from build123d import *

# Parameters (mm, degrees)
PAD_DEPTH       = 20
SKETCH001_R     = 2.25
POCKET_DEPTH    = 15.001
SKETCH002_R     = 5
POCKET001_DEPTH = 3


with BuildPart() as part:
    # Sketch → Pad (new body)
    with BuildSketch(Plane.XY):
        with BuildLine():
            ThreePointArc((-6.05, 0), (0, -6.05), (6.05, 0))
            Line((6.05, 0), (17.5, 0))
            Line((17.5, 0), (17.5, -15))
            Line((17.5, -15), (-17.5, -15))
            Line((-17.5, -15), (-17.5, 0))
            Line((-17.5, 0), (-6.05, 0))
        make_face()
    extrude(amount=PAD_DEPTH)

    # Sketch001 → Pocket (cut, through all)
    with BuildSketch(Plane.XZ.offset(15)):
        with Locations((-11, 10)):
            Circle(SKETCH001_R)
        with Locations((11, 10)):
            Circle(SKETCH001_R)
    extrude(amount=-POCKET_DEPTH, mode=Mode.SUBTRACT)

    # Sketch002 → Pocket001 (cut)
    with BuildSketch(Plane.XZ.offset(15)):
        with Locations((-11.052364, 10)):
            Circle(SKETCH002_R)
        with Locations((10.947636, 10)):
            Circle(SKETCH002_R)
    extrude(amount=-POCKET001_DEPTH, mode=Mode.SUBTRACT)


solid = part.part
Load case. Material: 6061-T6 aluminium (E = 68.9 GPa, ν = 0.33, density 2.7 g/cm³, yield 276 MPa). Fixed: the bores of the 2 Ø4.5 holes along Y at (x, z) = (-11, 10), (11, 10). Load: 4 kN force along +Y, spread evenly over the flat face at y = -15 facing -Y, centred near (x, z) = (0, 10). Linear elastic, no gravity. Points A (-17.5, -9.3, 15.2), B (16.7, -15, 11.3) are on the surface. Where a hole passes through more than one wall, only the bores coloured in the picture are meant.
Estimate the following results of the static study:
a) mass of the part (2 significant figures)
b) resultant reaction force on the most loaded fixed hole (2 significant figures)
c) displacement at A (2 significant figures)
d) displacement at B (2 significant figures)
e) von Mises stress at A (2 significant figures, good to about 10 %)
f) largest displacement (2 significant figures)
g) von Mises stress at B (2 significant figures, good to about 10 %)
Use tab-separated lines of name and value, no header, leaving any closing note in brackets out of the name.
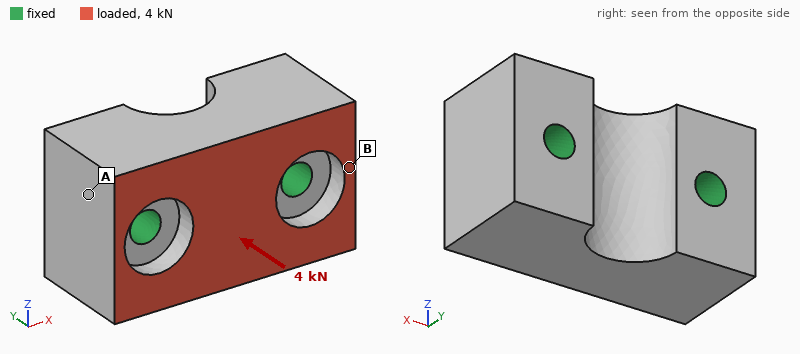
mass of the part	23 g
resultant reaction force on the most loaded fixed hole	2.0 kN
displacement at A	1.2 µm
displacement at B	1.4 µm
von Mises stress at A	6.7 MPa
largest displacement	3.8 µm
von Mises stress at B	16 MPa
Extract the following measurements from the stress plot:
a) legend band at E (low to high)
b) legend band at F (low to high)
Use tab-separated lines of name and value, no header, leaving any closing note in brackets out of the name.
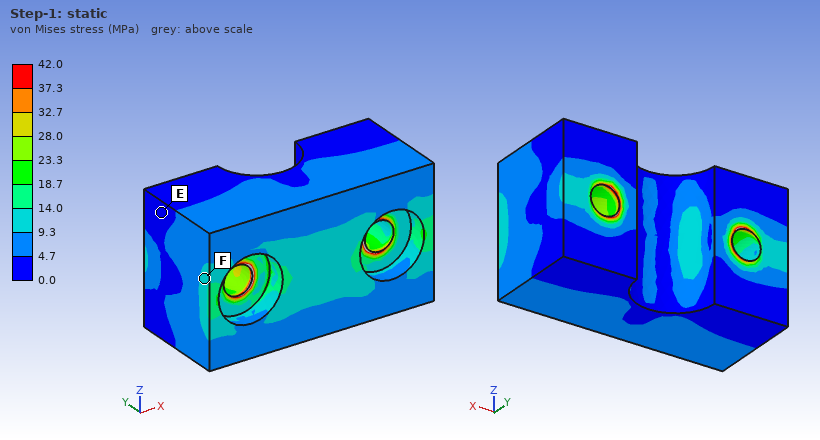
legend band at E	0.0 to 4.7 MPa
legend band at F	9.3 to 14.0 MPa
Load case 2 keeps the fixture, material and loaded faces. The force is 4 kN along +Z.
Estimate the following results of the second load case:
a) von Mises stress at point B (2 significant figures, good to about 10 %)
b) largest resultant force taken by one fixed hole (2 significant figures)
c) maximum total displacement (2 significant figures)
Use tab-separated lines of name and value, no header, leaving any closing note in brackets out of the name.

von Mises stress at point B	16 MPa
largest resultant force taken by one fixed hole	2.0 kN
maximum total displacement	11 µm
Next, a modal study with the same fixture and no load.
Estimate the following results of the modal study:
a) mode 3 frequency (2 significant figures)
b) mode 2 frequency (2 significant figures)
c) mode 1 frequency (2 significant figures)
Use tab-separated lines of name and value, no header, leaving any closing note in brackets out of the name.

mode 3 frequency	50 kHz
mode 2 frequency	49 kHz
mode 1 frequency	39 kHz
